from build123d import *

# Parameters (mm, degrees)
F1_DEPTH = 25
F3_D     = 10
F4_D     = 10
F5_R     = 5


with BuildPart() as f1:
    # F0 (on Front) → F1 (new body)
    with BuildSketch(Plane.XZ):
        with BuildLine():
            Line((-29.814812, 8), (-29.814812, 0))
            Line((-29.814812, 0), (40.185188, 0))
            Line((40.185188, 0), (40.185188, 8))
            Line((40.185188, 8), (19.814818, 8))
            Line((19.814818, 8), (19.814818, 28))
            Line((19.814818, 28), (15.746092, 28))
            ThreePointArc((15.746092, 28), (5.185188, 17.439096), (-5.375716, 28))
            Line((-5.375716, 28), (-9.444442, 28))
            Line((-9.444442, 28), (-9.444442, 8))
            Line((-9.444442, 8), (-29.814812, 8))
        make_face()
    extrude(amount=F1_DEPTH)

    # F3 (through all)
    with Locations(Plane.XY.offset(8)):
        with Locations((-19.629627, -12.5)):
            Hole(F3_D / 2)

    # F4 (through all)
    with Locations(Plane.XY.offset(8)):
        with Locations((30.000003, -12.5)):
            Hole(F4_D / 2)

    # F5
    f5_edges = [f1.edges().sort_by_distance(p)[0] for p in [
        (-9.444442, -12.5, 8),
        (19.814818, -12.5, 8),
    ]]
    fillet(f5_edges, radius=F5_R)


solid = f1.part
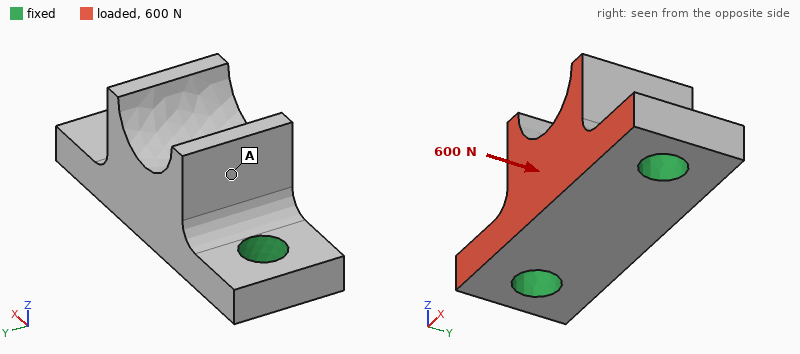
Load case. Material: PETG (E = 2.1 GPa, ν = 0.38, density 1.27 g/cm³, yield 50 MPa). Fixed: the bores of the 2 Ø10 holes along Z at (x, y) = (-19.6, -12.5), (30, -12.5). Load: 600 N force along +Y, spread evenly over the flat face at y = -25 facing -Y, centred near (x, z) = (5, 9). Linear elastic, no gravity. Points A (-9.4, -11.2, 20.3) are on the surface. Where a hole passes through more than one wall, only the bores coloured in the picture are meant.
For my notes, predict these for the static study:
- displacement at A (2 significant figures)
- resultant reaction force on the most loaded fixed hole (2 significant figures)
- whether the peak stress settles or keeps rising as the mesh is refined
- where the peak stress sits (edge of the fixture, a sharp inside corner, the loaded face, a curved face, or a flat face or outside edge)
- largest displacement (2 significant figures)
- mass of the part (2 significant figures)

0.076 mm
300 N
keeps rising
edge of the fixture
0.12 mm
30 g
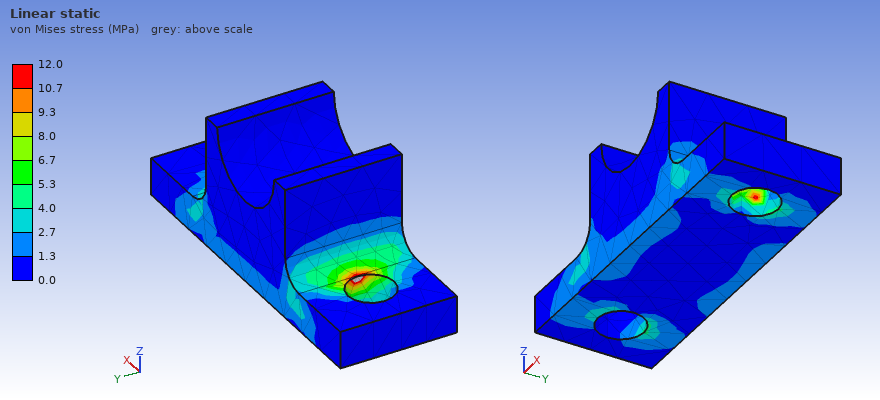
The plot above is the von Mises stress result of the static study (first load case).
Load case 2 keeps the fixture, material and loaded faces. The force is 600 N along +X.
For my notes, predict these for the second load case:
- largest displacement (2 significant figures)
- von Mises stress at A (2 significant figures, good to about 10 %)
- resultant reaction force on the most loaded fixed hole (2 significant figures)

56 µm
0.71 MPa
330 N
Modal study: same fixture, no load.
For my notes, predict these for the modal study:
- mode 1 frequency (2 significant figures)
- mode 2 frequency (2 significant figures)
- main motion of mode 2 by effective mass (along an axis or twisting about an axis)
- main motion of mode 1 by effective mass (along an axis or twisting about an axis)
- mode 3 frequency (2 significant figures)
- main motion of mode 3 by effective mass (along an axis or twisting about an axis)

2500 Hz
4300 Hz
along Z
along Y
5700 Hz
along X
